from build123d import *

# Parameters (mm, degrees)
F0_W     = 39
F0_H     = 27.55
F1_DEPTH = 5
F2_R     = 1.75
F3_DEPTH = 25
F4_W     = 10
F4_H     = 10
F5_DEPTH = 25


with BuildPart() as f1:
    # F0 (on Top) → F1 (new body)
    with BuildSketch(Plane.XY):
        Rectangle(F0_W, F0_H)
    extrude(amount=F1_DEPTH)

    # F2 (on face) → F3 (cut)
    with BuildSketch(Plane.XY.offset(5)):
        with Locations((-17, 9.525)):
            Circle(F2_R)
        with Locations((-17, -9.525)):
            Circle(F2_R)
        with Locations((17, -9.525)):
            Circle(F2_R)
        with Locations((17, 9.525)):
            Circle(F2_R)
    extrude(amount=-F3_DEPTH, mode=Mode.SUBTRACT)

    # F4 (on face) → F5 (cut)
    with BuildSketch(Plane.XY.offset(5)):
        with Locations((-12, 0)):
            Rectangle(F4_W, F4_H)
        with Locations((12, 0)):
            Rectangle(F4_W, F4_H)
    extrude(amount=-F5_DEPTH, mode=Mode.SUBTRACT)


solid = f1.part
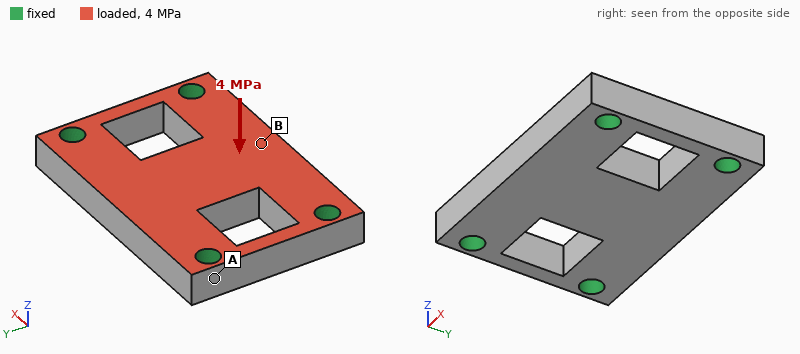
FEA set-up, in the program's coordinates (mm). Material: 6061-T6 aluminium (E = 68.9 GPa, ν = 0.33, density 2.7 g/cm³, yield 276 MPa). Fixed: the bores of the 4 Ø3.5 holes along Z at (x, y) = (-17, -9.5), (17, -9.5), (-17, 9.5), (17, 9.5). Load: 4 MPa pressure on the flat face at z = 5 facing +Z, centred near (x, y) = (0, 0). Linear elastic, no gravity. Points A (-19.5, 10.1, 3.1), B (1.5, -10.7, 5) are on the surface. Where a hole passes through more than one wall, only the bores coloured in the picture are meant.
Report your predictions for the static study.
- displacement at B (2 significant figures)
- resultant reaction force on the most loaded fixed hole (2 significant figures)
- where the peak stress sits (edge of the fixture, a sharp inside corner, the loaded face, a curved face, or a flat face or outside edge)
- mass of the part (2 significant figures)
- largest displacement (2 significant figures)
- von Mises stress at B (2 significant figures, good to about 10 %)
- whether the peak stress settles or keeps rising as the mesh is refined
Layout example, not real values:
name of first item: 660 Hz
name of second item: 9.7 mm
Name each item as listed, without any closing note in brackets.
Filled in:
displacement at B: 25 µm
resultant reaction force on the most loaded fixed hole: 840 N
where the peak stress sits: edge of the fixture
mass of the part: 11 g
largest displacement: 27 µm
von Mises stress at B: 47 MPa
whether the peak stress settles or keeps rising as the mesh is refined: keeps rising
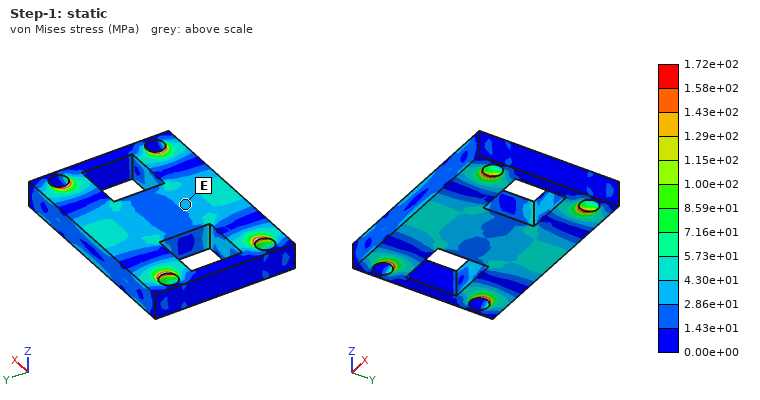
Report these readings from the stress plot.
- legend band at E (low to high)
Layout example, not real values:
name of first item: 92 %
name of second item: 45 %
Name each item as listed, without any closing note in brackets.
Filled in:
legend band at E: 2.86e+01 to 4.30e+01 MPa
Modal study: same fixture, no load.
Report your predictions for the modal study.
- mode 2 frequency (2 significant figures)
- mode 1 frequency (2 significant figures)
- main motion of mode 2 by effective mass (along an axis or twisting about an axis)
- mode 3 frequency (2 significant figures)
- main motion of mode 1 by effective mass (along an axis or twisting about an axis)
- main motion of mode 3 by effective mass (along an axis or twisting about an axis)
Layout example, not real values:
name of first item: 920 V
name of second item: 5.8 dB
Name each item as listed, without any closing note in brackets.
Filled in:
mode 2 frequency: 24 kHz
mode 1 frequency: 18 kHz
main motion of mode 2 by effective mass: twisting about X
mode 3 frequency: 25 kHz
main motion of mode 1 by effective mass: along Z
main motion of mode 3 by effective mass: along Y
